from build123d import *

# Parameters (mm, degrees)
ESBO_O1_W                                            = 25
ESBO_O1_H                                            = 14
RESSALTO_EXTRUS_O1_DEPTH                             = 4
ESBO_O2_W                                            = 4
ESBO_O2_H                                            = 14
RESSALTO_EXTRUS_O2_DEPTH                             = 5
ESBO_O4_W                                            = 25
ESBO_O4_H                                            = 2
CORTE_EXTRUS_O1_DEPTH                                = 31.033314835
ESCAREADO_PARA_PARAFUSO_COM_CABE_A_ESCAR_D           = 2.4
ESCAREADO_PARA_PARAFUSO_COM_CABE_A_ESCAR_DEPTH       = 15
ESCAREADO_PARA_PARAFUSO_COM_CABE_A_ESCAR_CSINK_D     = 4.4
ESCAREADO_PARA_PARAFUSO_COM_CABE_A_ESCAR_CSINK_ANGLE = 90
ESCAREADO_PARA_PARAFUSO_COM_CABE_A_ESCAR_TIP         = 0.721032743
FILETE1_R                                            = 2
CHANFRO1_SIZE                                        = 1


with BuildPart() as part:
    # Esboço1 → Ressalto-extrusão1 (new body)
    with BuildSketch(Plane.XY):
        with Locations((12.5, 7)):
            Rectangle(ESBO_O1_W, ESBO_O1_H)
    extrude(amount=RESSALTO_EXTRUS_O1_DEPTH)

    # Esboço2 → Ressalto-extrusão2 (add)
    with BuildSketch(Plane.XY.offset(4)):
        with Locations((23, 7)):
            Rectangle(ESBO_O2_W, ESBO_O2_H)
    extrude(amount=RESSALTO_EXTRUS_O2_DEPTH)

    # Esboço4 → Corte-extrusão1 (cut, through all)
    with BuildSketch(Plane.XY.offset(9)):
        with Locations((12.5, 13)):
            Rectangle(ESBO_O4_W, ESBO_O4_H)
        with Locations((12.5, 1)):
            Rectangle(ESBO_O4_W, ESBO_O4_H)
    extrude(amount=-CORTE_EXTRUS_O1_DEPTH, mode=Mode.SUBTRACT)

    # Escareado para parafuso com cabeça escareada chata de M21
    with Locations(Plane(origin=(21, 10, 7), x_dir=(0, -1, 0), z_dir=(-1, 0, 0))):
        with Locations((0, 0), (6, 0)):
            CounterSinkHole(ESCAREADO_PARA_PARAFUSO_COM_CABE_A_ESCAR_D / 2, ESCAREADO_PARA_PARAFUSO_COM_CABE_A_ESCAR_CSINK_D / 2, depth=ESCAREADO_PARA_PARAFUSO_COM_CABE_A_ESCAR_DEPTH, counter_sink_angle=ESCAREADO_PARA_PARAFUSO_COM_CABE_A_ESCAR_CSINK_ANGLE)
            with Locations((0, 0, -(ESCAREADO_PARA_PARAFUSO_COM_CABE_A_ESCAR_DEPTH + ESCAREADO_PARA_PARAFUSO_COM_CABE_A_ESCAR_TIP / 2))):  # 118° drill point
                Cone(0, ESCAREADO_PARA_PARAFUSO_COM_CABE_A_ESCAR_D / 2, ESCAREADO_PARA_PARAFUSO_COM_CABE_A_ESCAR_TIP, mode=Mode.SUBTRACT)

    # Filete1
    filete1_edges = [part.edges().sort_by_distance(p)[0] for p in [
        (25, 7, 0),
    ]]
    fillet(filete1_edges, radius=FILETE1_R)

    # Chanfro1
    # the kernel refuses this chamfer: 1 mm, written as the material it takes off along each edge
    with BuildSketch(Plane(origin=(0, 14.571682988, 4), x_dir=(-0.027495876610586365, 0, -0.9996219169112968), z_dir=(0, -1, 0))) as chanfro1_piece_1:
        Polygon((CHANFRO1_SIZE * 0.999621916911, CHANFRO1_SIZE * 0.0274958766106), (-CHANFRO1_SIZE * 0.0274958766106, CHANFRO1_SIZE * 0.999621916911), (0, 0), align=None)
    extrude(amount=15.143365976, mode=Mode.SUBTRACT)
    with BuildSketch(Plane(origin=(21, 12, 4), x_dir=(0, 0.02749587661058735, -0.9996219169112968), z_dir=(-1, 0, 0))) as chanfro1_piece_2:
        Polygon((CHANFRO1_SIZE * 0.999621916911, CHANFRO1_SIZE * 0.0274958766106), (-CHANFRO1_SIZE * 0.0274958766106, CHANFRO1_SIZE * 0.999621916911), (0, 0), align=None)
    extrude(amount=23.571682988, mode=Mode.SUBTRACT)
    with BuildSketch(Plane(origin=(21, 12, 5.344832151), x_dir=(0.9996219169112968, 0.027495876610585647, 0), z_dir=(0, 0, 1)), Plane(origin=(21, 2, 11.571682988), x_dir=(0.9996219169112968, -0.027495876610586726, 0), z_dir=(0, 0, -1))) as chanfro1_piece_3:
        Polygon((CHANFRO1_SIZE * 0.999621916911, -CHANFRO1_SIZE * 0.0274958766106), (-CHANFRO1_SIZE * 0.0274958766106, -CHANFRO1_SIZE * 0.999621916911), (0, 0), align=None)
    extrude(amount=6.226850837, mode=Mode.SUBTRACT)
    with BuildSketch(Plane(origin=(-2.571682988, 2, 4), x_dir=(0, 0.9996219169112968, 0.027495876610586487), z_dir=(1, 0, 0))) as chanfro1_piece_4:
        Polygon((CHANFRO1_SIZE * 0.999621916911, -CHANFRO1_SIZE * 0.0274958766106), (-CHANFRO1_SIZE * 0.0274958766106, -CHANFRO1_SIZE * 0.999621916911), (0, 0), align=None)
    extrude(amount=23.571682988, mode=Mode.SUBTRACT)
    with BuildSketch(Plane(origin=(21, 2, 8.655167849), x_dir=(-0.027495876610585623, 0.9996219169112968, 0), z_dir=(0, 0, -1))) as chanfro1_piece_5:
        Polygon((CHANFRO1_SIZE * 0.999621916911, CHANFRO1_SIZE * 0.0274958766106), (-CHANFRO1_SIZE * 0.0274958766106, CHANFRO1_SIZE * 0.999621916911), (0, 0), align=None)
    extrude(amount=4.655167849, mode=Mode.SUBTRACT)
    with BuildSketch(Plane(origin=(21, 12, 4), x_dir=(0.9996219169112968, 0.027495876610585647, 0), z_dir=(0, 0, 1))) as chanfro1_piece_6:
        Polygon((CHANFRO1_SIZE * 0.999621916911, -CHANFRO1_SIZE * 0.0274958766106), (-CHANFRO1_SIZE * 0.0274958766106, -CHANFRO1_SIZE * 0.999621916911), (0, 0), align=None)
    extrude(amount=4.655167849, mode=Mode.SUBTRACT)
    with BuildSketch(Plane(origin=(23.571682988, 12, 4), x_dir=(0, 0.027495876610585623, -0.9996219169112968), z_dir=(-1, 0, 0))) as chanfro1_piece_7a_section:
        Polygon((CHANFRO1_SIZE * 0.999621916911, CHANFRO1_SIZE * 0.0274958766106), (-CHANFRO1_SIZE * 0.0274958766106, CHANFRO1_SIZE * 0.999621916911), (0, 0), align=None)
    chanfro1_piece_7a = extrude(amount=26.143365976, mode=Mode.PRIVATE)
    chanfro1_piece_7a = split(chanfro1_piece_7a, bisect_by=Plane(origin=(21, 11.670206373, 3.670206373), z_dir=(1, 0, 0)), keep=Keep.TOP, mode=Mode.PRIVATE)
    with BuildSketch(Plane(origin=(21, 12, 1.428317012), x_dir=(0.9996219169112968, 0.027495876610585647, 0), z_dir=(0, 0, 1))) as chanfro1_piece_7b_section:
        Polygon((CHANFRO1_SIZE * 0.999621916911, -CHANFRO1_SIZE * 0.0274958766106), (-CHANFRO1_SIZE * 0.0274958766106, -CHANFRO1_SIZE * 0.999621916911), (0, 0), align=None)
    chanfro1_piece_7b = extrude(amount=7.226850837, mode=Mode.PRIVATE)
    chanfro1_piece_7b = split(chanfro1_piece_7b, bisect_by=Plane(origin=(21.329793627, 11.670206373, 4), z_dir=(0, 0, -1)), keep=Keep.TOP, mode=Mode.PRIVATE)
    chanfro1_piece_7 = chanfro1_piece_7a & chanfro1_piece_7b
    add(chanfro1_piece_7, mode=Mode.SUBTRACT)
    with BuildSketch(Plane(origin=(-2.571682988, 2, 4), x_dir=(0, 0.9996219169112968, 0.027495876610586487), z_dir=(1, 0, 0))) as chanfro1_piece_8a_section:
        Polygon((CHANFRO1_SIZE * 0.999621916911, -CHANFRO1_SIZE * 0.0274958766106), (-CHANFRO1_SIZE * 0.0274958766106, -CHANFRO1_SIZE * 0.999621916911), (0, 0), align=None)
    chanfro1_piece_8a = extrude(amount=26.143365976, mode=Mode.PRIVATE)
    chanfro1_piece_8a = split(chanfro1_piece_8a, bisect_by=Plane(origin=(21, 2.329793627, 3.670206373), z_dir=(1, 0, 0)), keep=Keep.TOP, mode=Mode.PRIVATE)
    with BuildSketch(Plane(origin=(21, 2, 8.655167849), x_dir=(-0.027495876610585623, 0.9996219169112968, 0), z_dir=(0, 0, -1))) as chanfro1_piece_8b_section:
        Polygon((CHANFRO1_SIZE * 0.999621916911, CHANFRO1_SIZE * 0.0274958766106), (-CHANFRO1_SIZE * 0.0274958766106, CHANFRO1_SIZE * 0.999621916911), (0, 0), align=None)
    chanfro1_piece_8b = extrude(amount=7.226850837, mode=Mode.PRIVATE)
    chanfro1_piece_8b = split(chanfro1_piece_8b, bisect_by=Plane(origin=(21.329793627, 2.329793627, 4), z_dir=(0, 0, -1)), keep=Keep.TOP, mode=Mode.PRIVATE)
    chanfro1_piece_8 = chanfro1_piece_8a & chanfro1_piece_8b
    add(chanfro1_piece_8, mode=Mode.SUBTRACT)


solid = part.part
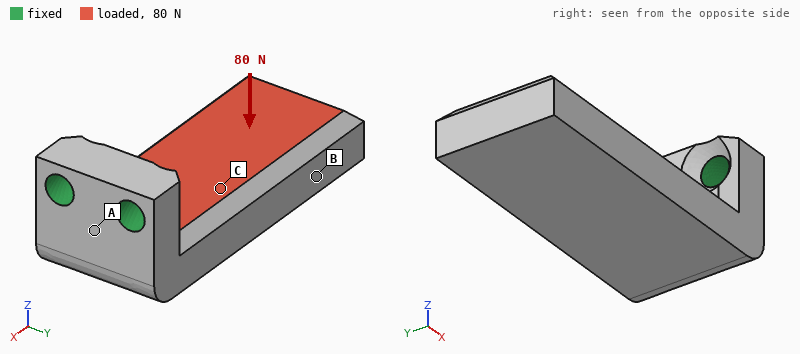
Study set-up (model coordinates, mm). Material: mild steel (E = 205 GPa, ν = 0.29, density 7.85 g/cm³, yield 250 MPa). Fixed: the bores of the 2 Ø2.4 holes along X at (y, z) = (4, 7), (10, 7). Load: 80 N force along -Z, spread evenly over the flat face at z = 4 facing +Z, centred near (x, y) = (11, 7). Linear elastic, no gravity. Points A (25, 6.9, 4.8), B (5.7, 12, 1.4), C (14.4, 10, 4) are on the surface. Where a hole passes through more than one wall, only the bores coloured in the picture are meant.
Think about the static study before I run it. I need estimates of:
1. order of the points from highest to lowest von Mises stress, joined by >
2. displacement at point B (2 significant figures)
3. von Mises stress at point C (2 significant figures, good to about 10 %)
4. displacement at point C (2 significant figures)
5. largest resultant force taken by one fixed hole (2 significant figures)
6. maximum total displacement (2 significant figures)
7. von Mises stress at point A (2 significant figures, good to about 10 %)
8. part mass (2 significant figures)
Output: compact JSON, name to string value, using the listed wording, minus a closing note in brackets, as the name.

{"order of the points from highest to lowest von Mises stress, joined by >": "A > C > B", "displacement at point B": "15 µm", "von Mises stress at point C": "15 MPa", "displacement at point C": "6.1 µm", "largest resultant force taken by one fixed hole": "43 N", "maximum total displacement": "21 µm", "von Mises stress at point A": "28 MPa", "part mass": "8.8 g"}
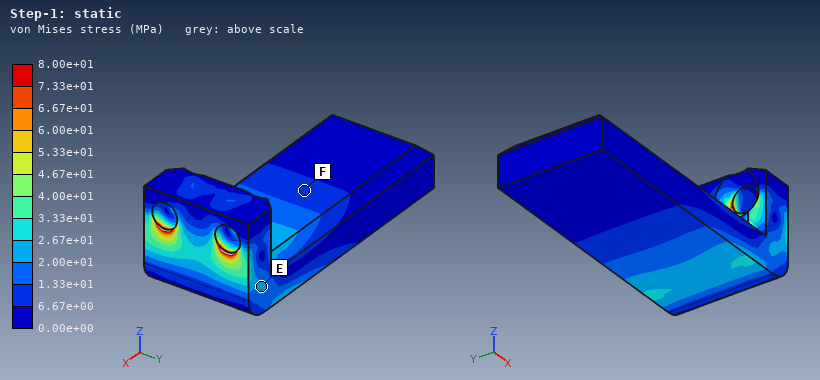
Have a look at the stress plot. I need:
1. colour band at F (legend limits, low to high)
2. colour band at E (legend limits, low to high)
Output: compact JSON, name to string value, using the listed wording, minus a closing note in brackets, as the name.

{"colour band at F": "6.67e+00 to 1.33e+01 MPa", "colour band at E": "2.00e+01 to 2.67e+01 MPa"}
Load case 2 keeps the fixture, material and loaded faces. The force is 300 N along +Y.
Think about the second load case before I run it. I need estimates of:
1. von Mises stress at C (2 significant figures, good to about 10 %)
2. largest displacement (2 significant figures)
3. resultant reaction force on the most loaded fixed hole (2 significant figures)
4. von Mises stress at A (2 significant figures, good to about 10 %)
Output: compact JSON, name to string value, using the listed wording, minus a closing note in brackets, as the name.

{"von Mises stress at C": "29 MPa", "largest displacement": "26 µm", "resultant reaction force on the most loaded fixed hole": "510 N", "von Mises stress at A": "59 MPa"}
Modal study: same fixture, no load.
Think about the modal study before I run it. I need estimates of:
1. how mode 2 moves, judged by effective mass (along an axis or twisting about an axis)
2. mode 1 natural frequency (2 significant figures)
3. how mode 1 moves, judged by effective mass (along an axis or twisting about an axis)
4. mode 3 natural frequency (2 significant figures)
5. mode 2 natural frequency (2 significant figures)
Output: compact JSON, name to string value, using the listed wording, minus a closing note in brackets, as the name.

{"how mode 2 moves, judged by effective mass": "along Y", "mode 1 natural frequency": "4600 Hz", "how mode 1 moves, judged by effective mass": "along Z", "mode 3 natural frequency": "24 kHz", "mode 2 natural frequency": "8400 Hz"}
